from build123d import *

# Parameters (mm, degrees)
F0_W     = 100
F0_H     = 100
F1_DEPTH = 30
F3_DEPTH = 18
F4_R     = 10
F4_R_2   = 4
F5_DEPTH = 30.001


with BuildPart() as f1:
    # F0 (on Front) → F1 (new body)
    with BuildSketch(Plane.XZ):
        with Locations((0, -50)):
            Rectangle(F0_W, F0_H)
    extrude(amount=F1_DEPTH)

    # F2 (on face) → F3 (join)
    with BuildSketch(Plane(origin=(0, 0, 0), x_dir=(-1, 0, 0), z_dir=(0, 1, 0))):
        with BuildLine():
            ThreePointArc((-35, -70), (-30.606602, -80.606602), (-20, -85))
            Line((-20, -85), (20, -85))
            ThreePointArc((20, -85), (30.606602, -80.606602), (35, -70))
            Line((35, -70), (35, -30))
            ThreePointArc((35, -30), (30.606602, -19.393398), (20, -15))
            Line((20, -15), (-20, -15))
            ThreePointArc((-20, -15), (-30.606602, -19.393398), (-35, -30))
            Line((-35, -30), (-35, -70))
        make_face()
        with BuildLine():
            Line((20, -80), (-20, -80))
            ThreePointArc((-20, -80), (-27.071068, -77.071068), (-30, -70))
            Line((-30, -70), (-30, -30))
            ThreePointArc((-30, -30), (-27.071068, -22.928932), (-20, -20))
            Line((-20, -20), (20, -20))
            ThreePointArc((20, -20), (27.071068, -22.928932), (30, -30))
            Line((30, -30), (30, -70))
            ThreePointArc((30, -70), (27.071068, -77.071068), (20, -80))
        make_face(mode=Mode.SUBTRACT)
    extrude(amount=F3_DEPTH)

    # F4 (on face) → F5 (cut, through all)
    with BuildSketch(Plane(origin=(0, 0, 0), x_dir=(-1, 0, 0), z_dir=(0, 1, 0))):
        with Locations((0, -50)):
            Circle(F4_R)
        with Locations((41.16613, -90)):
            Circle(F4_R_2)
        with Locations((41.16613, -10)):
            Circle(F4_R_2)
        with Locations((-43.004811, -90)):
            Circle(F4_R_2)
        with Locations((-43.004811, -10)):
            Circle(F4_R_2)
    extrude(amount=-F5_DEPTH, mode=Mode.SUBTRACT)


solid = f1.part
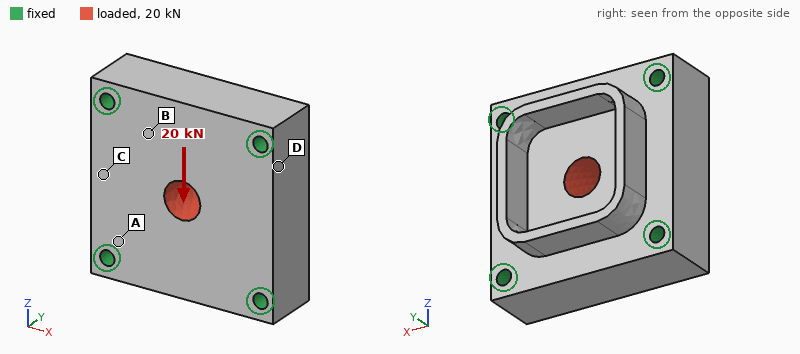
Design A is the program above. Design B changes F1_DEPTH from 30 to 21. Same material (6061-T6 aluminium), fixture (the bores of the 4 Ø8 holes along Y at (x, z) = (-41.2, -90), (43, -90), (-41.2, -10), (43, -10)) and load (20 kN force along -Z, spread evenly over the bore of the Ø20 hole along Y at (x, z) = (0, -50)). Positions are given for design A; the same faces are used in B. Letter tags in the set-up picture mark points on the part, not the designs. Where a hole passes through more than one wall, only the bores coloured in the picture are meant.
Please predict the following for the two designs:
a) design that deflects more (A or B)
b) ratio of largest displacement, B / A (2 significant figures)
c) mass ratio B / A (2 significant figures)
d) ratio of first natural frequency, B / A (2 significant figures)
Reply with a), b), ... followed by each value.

a) B
b) 1.4
c) 0.72
d) 0.85
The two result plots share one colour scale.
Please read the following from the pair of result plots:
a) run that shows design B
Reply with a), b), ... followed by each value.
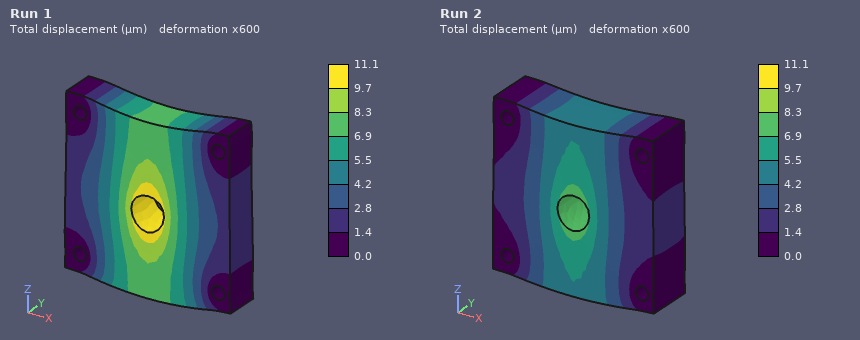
a) Run 1
